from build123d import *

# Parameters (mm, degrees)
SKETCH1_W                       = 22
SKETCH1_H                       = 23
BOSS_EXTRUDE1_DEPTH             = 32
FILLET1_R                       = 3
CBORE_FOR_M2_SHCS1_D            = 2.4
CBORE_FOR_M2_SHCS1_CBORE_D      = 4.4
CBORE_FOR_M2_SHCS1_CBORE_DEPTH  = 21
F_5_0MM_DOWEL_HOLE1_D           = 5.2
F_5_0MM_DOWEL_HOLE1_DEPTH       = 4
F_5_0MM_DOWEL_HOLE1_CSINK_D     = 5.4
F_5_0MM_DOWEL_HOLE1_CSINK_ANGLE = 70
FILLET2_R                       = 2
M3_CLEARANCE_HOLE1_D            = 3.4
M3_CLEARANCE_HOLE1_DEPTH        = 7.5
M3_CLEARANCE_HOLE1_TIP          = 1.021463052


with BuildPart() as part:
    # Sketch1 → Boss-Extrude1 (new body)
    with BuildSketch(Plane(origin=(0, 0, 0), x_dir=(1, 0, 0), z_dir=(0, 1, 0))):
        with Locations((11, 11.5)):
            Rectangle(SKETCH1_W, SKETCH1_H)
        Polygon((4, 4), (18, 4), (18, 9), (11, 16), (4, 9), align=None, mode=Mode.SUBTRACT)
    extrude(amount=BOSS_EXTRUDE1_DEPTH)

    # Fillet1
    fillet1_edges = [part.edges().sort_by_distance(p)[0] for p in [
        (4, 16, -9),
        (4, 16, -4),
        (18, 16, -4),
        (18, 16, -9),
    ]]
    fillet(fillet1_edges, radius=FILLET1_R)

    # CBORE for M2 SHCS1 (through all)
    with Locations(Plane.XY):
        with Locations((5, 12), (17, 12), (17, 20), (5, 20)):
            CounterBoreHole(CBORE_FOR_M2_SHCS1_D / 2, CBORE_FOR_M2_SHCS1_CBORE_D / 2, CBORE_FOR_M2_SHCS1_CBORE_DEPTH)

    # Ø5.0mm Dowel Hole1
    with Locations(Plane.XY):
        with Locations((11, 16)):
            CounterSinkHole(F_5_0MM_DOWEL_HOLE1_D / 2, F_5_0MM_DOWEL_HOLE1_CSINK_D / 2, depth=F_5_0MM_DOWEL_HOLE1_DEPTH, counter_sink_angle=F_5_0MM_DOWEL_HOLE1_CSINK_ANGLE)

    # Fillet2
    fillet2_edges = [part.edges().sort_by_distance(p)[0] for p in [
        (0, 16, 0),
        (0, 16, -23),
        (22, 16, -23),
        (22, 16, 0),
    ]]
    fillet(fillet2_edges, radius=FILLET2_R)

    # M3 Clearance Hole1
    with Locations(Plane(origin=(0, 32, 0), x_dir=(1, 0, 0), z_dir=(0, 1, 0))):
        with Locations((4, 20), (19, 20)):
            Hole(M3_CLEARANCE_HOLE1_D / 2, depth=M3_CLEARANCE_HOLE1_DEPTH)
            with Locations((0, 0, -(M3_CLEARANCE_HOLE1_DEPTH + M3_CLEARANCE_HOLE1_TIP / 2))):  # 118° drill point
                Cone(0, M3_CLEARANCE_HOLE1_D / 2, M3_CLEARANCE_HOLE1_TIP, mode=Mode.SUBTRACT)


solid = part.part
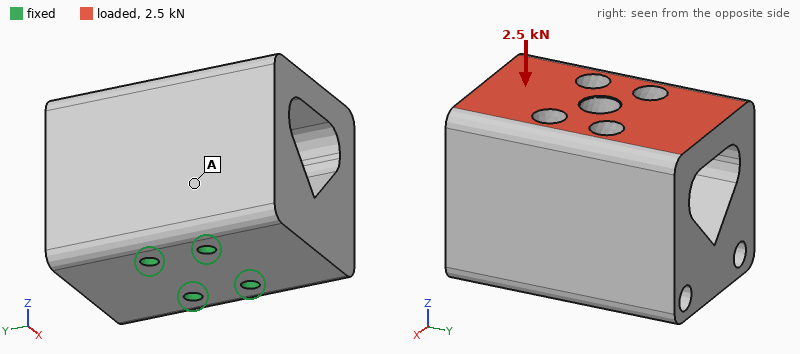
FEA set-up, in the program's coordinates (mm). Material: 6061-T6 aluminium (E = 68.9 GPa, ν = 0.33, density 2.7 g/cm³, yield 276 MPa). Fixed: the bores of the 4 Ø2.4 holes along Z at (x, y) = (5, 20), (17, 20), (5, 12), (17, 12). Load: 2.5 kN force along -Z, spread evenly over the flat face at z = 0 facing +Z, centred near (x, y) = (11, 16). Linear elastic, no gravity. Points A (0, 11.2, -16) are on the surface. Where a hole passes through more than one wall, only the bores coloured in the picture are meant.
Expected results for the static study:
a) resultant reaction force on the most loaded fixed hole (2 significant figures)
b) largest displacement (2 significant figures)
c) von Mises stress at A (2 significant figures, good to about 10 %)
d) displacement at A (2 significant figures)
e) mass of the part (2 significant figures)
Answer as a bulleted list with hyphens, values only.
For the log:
- 640 N
- 15 µm
- 13 MPa
- 4.9 µm
- 30 g
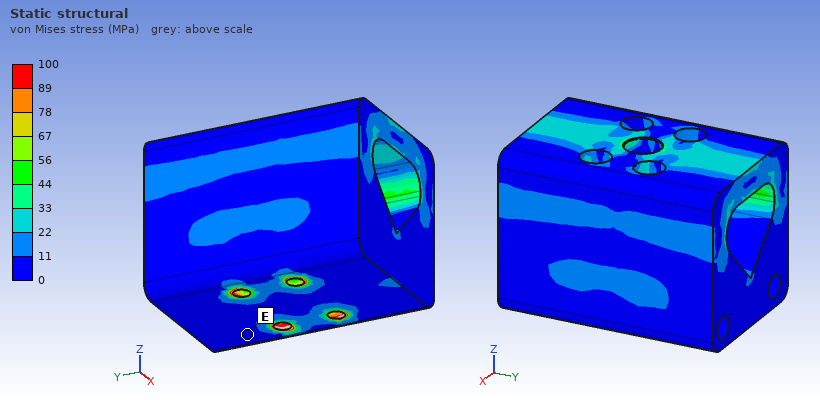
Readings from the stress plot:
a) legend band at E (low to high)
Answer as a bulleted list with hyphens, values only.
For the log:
- 0 to 11 MPa
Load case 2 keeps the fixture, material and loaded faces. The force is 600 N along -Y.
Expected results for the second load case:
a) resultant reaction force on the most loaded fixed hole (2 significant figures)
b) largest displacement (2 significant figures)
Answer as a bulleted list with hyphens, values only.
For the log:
- 700 N
- 30 µm
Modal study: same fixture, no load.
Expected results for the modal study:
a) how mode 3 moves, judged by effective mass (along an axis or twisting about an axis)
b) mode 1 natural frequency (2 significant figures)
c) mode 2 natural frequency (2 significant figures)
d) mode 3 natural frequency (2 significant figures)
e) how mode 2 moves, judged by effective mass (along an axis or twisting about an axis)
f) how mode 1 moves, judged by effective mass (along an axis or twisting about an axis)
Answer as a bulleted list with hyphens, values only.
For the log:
- twisting about Z
- 6900 Hz
- 9700 Hz
- 17 kHz
- along X
- along Y
